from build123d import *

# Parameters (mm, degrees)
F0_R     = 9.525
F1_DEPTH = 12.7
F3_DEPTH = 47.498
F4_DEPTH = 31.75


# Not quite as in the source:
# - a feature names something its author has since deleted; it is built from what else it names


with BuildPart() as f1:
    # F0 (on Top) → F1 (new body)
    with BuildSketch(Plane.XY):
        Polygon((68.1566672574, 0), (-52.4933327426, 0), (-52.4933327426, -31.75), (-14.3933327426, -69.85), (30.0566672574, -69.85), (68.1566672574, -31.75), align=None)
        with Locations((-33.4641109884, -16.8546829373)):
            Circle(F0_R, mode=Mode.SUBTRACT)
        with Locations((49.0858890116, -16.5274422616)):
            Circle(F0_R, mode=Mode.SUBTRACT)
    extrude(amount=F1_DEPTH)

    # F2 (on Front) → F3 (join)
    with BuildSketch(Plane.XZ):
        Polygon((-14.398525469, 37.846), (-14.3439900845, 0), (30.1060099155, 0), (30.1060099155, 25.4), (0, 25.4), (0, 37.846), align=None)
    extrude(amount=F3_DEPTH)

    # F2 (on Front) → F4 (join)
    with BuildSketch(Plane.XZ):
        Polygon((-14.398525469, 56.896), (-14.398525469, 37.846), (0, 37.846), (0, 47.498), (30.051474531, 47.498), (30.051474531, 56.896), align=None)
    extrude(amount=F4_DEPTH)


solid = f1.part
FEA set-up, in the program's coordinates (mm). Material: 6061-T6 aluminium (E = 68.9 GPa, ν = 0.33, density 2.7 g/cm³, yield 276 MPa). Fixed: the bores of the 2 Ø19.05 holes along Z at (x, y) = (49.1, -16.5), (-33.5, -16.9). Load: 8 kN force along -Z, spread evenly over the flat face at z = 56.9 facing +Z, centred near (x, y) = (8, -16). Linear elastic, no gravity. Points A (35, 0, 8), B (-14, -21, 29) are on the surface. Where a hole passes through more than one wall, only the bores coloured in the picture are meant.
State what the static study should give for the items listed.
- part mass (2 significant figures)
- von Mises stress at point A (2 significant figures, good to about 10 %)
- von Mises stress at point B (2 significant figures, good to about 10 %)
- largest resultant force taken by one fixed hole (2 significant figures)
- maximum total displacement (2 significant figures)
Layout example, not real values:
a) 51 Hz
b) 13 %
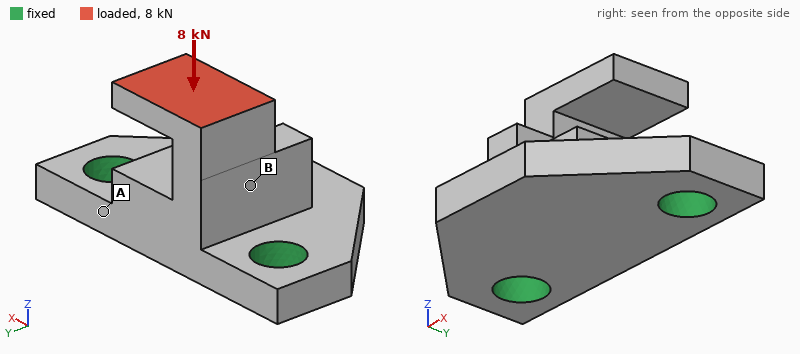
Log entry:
a) 360 g
b) 23 MPa
c) 70 MPa
d) 4.7 kN
e) 0.49 mm
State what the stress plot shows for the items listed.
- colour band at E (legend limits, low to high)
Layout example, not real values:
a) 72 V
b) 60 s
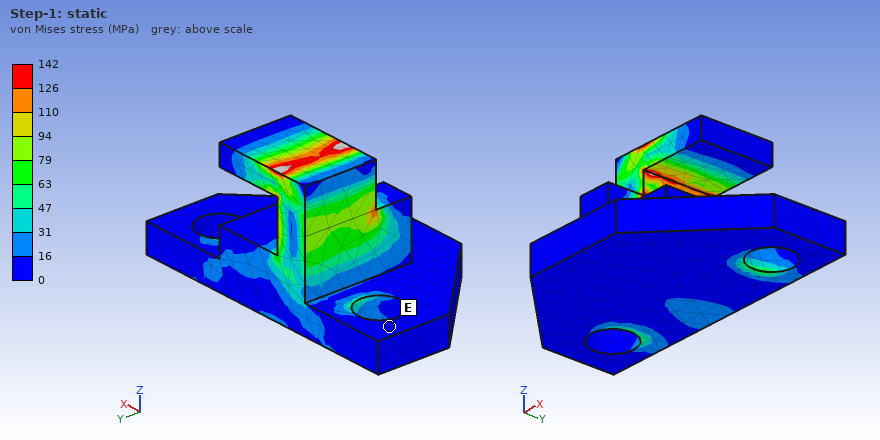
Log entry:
a) 0 to 16 MPa
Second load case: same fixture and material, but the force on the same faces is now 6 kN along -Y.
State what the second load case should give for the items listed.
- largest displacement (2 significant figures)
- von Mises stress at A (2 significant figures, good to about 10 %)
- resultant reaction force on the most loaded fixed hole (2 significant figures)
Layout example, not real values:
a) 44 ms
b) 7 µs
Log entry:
a) 0.34 mm
b) 72 MPa
c) 3.5 kN
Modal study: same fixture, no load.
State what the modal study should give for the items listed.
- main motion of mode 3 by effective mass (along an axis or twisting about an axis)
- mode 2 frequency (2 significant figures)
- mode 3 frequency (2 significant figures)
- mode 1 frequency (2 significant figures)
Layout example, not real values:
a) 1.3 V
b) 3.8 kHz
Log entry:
a) along Z
b) 3600 Hz
c) 5800 Hz
d) 3300 Hz
